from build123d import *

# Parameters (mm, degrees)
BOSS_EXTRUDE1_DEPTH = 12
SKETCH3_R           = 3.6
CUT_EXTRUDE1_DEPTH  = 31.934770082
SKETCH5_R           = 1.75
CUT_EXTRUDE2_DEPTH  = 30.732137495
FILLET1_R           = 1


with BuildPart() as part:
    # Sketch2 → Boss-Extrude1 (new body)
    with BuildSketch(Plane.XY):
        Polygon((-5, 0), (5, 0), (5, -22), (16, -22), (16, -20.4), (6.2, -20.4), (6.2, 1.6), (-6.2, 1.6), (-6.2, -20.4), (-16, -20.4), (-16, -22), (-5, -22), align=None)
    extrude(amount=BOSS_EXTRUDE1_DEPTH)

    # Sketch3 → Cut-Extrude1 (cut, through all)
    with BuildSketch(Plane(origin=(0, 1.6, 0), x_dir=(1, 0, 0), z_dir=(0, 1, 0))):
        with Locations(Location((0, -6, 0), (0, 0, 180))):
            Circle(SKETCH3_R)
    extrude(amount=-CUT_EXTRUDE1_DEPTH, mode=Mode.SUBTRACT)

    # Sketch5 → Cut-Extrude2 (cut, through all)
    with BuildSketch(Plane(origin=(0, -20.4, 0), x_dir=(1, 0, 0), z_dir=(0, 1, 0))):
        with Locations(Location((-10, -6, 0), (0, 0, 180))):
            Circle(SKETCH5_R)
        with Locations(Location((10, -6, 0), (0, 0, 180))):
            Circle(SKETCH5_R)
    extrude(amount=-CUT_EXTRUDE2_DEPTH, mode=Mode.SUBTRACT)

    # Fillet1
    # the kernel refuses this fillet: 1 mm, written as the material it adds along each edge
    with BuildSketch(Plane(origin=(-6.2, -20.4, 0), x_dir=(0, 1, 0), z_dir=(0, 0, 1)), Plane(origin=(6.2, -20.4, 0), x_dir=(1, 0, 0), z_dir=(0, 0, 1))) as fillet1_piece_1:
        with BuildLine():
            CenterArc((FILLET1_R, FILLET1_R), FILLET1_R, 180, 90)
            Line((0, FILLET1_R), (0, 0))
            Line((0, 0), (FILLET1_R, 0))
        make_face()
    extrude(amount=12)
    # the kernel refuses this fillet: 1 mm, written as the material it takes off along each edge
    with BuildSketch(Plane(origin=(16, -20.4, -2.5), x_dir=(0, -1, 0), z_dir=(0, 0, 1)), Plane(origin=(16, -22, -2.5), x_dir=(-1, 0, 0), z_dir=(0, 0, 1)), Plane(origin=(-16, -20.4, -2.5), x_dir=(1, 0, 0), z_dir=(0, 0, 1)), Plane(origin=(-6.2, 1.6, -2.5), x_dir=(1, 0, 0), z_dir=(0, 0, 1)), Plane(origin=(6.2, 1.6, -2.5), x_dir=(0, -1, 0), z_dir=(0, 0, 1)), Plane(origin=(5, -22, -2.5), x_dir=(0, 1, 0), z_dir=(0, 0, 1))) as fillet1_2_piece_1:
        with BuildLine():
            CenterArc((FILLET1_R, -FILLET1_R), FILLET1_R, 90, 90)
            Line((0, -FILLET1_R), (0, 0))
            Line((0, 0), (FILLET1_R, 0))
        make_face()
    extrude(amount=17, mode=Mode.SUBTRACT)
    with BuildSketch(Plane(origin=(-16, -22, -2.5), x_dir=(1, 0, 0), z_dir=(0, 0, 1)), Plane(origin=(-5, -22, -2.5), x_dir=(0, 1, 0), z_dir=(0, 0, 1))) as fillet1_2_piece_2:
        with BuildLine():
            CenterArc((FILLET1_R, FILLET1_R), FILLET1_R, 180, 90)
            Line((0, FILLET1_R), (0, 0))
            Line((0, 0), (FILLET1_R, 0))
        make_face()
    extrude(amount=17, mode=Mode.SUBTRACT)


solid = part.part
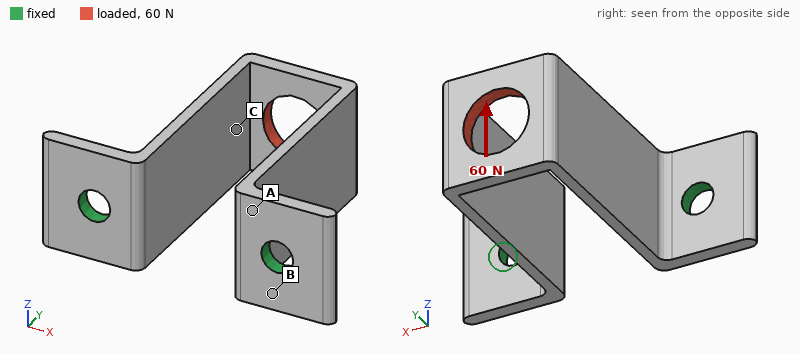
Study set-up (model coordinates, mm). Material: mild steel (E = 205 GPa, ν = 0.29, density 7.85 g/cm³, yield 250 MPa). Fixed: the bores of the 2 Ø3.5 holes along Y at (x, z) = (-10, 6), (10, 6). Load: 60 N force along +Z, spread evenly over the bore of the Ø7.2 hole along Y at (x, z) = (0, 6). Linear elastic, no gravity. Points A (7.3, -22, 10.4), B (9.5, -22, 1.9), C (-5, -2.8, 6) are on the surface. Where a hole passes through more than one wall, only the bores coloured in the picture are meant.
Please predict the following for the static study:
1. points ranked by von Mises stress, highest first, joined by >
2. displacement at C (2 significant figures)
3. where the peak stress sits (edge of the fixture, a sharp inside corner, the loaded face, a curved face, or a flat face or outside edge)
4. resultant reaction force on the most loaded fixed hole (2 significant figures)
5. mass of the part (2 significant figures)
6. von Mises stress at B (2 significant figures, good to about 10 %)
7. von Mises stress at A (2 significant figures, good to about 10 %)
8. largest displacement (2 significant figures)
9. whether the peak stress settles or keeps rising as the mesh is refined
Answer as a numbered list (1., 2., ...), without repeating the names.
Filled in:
1. B > A > C
2. 24 µm
3. edge of the fixture
4. 30 N
5. 8.9 g
6. 47 MPa
7. 29 MPa
8. 32 µm
9. keeps rising
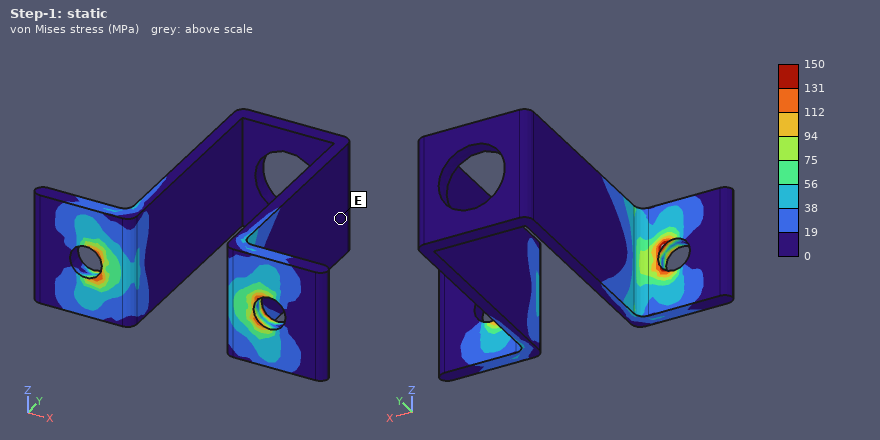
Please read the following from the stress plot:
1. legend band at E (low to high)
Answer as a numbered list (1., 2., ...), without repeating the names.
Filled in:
1. 0 to 19 MPa
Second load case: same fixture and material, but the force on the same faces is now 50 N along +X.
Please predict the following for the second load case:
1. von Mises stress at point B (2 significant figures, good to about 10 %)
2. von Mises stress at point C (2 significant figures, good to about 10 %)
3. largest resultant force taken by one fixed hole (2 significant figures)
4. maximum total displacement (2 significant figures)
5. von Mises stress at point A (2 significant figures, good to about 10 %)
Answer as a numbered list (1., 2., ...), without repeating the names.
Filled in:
1. 12 MPa
2. 57 MPa
3. 54 N
4. 66 µm
5. 29 MPa
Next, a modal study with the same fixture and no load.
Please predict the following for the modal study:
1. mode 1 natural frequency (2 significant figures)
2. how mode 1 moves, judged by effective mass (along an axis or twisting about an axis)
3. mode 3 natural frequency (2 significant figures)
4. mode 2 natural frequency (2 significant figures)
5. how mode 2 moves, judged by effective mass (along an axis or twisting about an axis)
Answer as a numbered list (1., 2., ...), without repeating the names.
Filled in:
1. 2500 Hz
2. along X
3. 5500 Hz
4. 4200 Hz
5. along Z
